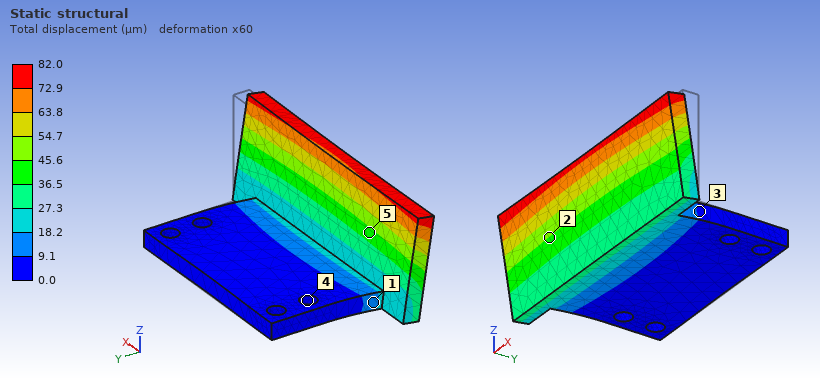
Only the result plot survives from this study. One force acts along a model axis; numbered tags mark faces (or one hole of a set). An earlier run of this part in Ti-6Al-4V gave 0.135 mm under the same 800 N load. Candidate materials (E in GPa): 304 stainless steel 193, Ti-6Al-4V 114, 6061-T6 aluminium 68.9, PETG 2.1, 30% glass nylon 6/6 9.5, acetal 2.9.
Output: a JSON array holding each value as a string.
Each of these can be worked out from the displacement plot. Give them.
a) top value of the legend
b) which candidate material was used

["82.0 µm", "304 stainless steel"]
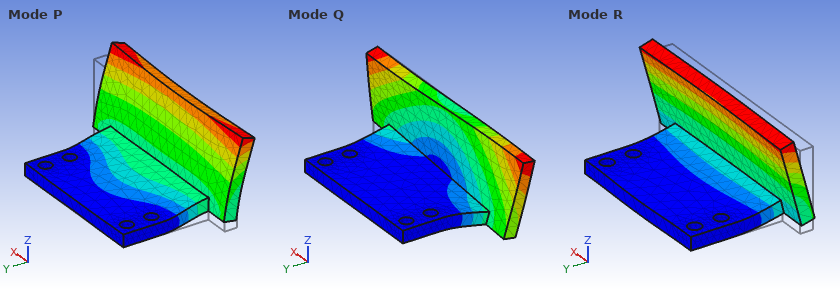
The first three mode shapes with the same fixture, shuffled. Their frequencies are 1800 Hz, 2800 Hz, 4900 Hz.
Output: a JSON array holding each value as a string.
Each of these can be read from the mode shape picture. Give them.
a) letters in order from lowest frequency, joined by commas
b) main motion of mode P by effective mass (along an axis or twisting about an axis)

["R, Q, P", "along Z"]
